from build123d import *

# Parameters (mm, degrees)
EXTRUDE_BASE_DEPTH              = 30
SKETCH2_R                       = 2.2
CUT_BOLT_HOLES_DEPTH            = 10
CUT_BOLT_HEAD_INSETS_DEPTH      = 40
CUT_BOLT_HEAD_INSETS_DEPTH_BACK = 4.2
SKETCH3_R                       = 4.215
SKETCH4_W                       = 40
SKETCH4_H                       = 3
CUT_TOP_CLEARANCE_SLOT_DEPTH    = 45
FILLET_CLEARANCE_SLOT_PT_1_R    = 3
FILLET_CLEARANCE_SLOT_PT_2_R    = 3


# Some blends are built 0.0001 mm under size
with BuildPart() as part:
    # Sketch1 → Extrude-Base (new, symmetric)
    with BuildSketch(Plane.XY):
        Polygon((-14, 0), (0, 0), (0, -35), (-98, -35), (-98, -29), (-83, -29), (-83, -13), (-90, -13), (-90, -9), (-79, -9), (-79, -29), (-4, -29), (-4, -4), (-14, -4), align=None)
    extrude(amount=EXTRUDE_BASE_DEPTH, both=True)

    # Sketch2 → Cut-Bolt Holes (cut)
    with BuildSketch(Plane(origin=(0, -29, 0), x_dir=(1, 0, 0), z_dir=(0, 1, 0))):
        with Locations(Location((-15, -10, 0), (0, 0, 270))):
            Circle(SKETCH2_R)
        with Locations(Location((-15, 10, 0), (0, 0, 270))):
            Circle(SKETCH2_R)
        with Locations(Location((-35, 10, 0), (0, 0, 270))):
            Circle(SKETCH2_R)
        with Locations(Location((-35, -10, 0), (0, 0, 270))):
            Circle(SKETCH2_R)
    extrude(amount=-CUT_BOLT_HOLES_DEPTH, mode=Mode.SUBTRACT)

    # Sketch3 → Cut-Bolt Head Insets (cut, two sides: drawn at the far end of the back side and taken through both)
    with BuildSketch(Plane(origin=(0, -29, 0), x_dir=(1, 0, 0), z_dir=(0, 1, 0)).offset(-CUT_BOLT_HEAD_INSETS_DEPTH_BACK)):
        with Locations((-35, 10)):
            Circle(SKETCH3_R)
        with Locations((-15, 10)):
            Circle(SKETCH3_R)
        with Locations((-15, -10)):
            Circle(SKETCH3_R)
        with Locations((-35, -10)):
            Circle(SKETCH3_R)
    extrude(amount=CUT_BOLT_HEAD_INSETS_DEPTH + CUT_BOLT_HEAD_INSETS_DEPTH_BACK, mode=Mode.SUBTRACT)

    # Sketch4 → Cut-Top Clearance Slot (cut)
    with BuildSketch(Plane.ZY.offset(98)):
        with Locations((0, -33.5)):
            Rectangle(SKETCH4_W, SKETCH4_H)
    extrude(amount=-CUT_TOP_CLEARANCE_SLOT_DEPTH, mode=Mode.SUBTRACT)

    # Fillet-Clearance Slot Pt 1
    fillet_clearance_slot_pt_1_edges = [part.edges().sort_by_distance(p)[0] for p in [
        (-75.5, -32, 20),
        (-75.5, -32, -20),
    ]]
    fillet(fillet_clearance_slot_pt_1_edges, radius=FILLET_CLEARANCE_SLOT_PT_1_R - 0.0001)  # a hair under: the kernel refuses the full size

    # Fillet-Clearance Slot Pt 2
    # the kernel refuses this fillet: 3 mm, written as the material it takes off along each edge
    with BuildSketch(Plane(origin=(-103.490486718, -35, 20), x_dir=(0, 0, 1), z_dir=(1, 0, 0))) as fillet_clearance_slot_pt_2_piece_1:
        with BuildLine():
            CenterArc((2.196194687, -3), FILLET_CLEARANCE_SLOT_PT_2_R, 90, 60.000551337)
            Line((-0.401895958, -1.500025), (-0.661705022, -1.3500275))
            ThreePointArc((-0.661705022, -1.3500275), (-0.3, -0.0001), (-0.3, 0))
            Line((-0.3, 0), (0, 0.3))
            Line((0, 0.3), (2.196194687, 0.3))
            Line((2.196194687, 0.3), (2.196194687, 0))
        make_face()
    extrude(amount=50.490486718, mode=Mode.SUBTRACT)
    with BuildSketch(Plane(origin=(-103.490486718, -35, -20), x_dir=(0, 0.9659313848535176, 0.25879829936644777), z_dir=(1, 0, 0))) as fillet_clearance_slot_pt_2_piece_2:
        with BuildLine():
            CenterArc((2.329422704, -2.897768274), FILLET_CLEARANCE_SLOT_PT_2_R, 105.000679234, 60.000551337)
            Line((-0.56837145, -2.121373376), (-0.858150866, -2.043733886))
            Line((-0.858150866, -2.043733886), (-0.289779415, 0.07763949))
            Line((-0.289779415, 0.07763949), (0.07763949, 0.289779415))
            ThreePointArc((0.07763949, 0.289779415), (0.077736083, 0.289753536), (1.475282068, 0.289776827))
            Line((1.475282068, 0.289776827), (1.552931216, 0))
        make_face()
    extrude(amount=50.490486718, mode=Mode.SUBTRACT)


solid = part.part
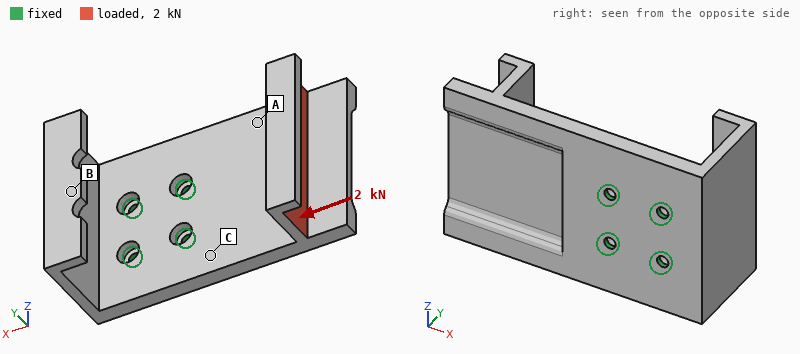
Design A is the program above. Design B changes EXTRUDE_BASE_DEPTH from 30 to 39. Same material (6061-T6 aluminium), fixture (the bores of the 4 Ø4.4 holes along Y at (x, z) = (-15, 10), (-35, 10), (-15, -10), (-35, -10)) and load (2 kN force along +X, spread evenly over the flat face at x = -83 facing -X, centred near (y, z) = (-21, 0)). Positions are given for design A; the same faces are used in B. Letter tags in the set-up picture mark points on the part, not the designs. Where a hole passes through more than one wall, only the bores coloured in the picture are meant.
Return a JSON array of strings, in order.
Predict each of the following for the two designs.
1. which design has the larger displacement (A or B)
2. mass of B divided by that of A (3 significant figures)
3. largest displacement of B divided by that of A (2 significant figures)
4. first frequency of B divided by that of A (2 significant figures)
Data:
["A", "1.34", "0.71", "0.98"]
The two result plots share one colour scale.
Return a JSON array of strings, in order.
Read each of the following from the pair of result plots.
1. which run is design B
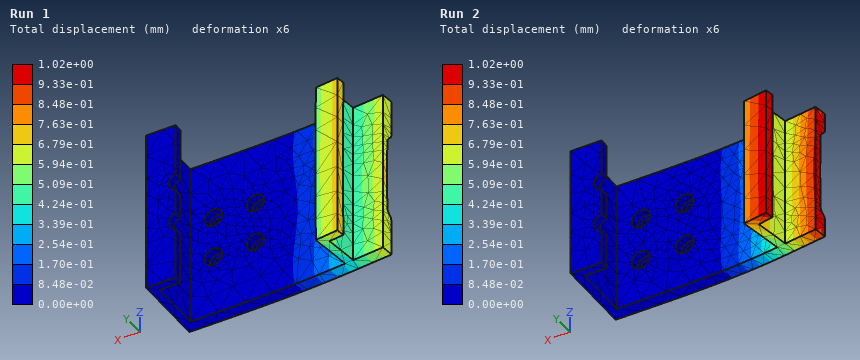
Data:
["Run 1"]
